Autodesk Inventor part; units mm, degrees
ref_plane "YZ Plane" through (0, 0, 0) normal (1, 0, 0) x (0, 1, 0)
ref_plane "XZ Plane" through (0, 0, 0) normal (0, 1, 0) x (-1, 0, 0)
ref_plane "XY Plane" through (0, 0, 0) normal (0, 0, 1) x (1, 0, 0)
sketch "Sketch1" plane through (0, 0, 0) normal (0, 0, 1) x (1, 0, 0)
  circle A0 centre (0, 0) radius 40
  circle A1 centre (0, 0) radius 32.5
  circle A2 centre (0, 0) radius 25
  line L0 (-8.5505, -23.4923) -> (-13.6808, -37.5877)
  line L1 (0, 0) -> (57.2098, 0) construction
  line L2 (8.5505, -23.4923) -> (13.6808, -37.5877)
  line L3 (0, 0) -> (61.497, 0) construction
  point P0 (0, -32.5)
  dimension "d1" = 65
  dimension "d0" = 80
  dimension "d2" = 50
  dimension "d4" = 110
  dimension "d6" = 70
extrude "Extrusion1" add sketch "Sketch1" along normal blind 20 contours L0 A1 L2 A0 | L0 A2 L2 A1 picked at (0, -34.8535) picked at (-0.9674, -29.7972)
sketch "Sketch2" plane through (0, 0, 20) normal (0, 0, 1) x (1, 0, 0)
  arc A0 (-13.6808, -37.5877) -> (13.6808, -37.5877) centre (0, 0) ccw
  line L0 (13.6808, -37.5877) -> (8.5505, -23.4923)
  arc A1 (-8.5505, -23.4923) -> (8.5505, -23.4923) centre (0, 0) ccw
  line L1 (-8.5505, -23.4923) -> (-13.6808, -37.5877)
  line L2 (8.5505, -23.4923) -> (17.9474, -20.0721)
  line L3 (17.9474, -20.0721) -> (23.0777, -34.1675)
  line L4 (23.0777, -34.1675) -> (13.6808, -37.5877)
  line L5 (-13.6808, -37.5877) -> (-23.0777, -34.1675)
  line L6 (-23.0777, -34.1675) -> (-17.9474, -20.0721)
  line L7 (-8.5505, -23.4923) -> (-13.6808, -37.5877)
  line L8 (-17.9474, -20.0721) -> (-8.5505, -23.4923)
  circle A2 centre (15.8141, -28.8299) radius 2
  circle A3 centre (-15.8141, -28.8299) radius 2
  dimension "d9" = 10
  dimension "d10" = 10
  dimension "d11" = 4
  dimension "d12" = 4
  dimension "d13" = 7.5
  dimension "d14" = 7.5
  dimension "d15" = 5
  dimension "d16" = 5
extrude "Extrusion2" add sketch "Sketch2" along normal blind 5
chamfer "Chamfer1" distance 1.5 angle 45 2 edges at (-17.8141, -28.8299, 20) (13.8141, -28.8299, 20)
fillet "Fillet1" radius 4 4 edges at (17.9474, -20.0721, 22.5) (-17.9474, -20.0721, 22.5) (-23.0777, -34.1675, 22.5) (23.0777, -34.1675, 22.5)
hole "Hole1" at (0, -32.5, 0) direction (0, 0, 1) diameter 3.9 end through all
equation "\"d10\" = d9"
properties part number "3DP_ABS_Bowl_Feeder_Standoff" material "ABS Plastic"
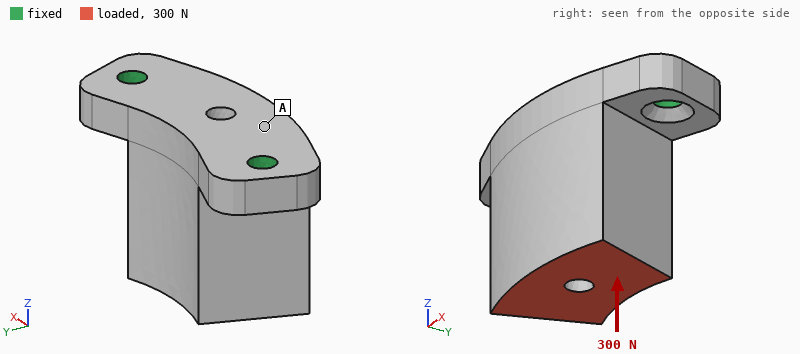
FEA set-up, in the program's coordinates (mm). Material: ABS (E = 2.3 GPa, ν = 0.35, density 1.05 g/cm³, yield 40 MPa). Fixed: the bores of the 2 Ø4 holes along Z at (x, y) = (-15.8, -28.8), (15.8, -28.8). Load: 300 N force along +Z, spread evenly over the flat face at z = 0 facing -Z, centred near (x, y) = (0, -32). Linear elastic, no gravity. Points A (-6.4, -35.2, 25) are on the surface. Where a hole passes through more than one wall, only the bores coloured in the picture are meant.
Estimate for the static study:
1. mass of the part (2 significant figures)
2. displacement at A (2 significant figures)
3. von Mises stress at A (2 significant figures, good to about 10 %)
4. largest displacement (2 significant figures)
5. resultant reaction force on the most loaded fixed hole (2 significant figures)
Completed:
10.0 g
0.077 mm
2.3 MPa
0.19 mm
160 N
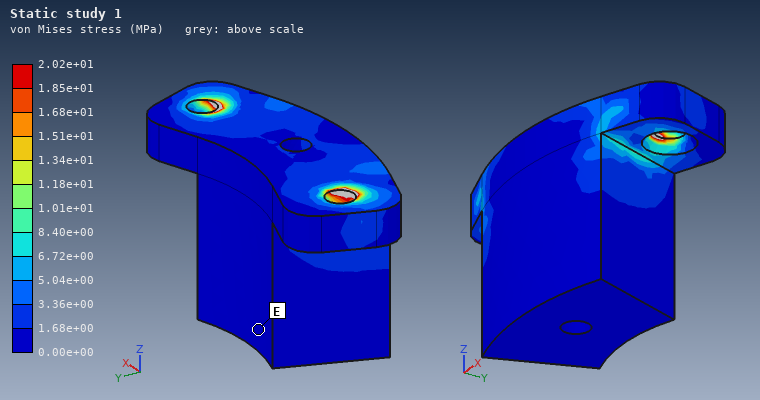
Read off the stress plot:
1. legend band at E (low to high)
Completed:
0.00e+00 to 1.68e+00 MPa
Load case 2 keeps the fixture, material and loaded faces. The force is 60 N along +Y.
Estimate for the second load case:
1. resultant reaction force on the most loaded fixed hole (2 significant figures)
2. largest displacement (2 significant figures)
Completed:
35 N
0.31 mm
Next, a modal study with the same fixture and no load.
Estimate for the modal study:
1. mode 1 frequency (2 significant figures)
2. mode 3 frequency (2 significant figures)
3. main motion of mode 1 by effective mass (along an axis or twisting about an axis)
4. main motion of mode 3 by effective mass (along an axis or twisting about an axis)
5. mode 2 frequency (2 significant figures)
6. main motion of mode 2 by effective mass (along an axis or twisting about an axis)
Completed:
1300 Hz
4600 Hz
along Y
along Z
4100 Hz
along X
